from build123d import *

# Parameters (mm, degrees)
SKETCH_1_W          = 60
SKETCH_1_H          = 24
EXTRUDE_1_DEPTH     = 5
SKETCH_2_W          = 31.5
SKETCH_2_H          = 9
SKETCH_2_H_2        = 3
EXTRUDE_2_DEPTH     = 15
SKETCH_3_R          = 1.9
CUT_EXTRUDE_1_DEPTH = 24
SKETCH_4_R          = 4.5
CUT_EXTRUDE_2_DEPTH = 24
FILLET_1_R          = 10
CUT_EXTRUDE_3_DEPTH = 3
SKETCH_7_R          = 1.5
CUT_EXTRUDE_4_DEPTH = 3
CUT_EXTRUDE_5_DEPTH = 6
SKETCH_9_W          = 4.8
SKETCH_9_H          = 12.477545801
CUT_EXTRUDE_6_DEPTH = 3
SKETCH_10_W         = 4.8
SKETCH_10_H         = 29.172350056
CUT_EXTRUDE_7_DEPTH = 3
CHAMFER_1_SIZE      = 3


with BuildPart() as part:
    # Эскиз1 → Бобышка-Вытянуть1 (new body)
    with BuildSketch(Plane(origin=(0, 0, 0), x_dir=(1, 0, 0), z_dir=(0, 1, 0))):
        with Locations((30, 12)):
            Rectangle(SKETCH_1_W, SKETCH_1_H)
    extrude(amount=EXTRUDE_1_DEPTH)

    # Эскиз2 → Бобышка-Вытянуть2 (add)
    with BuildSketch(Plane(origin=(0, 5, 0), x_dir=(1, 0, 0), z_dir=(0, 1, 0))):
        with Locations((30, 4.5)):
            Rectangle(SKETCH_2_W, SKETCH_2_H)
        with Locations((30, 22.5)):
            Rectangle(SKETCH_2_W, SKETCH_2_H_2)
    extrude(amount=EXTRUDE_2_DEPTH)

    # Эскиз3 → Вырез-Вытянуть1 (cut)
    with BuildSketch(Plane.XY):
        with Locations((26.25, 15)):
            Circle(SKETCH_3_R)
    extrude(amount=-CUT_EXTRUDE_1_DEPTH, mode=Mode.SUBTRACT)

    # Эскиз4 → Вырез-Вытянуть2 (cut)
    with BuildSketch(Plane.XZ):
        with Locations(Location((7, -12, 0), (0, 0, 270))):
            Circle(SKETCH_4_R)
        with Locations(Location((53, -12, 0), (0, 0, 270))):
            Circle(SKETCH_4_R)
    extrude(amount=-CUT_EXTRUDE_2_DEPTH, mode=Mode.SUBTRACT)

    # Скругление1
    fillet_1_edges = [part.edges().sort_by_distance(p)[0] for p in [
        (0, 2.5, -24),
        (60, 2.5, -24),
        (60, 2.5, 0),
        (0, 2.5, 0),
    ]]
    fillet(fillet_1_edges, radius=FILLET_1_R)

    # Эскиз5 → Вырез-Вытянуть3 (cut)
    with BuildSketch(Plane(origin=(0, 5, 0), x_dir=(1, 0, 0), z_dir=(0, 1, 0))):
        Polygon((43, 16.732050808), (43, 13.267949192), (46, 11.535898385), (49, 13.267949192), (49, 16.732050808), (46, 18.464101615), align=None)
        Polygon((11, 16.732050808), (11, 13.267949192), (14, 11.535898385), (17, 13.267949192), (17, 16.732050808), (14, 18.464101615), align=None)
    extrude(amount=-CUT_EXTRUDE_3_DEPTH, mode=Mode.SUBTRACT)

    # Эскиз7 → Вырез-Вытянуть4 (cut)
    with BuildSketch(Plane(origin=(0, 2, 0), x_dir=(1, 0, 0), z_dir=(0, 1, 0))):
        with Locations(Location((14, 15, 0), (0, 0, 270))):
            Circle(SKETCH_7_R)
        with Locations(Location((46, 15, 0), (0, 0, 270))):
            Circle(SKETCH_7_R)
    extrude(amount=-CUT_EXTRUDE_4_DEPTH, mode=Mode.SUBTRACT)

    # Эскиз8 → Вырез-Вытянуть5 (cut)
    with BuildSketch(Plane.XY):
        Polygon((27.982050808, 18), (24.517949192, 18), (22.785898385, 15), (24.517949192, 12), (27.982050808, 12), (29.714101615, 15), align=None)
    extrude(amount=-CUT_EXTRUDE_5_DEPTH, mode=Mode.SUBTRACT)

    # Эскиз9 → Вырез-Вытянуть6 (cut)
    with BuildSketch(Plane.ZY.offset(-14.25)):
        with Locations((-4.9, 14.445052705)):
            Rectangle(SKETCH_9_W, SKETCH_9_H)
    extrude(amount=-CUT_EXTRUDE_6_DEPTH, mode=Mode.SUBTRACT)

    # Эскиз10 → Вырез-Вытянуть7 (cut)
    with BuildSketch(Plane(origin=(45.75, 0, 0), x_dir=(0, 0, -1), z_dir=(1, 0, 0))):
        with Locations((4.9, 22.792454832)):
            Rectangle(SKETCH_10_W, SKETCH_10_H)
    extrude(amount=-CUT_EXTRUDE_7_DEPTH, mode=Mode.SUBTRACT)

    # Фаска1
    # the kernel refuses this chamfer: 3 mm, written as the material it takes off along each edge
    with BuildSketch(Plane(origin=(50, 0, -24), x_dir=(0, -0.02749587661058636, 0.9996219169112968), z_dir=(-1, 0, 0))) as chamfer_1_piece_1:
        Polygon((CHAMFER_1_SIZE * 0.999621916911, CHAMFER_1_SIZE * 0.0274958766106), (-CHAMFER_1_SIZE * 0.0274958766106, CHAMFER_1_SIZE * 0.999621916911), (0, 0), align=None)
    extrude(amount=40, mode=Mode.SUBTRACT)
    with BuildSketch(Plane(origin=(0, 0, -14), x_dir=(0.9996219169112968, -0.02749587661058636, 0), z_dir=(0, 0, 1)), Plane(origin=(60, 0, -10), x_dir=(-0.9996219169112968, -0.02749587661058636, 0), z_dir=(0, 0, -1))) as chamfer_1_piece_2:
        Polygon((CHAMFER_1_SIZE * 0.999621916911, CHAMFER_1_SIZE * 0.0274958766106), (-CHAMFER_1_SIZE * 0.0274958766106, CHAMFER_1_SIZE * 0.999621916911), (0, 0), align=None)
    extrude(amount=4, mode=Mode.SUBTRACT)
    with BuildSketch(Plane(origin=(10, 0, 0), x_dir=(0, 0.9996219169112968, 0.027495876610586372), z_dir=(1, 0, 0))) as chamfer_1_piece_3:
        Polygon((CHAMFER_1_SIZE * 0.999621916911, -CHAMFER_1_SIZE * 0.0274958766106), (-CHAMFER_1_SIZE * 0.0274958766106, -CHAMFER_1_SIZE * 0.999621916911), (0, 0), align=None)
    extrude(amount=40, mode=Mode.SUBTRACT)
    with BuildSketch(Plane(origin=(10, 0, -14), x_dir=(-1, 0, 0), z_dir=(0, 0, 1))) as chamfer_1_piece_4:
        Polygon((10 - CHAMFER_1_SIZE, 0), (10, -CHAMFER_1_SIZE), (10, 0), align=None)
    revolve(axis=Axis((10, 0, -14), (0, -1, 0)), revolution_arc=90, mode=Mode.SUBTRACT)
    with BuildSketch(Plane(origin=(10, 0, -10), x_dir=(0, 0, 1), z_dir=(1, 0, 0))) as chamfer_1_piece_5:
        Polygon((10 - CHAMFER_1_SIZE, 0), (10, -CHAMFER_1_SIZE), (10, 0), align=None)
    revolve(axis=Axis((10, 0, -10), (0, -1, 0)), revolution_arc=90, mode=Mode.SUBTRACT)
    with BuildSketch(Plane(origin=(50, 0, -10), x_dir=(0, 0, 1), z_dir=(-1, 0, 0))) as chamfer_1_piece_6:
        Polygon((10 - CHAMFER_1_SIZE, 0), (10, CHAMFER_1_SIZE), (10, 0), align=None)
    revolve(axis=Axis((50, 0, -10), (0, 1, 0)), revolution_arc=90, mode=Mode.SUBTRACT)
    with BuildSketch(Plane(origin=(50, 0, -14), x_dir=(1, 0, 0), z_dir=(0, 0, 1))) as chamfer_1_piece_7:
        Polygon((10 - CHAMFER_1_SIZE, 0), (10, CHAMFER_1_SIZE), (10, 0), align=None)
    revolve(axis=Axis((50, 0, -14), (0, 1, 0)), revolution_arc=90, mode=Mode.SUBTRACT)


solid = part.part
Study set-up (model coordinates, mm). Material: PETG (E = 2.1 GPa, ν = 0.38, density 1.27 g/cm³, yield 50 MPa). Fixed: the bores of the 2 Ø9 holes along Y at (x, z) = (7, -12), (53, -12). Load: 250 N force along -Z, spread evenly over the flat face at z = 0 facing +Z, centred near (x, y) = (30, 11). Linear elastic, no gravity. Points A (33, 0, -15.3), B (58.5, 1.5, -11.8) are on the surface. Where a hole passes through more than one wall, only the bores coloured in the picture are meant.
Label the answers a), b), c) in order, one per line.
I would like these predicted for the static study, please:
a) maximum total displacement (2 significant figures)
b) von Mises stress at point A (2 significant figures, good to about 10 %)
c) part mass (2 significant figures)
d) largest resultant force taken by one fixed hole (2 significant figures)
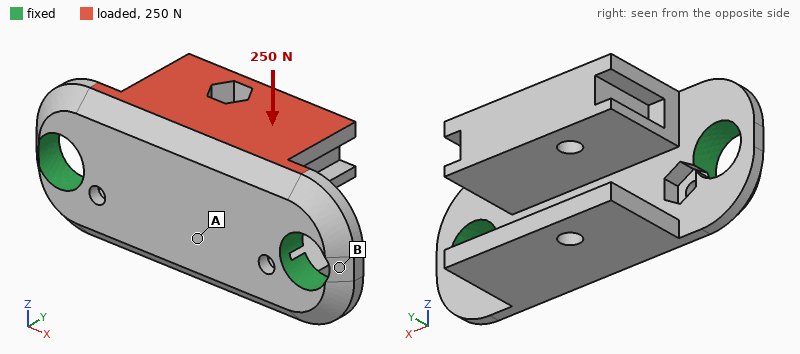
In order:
a) 0.39 mm
b) 3.2 MPa
c) 13 g
d) 130 N
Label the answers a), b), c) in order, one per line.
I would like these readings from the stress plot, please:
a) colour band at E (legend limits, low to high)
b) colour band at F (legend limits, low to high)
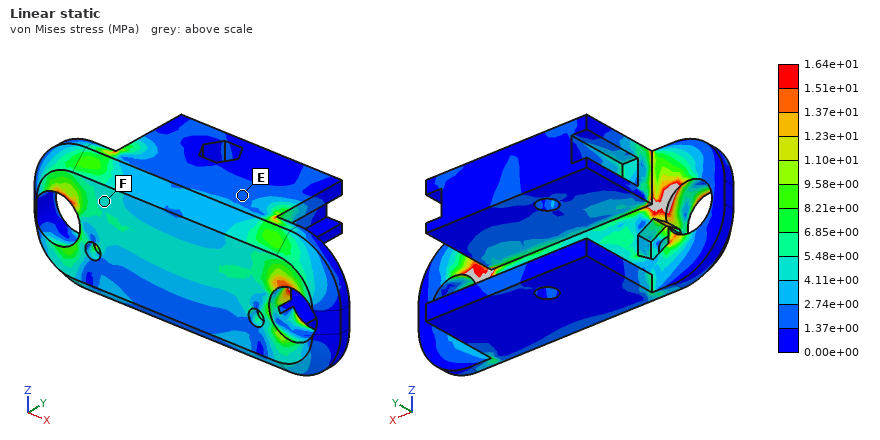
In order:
a) 1.37e+00 to 2.74e+00 MPa
b) 4.11e+00 to 5.48e+00 MPa
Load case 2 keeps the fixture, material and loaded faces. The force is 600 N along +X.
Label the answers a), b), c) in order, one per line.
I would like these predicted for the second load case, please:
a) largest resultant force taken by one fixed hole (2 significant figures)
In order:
a) 360 N
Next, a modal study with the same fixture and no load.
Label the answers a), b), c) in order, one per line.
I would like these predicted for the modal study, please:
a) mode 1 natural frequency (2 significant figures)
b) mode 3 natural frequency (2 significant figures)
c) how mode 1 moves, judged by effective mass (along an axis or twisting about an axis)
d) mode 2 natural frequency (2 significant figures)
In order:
a) 1700 Hz
b) 3000 Hz
c) along Z
d) 2200 Hz
